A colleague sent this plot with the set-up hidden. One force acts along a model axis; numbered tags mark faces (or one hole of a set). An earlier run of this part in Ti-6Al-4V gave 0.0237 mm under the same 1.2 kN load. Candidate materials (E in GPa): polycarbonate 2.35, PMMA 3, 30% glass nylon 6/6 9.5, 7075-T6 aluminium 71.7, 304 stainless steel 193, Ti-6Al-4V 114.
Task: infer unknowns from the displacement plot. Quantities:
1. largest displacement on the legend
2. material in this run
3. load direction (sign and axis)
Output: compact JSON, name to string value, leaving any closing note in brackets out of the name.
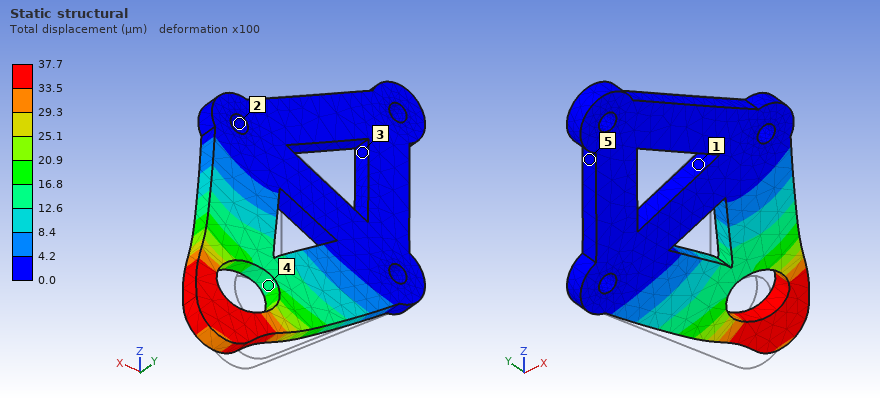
{"largest displacement on the legend": "37.7 µm", "material in this run": "7075-T6 aluminium", "load direction": "+X"}
